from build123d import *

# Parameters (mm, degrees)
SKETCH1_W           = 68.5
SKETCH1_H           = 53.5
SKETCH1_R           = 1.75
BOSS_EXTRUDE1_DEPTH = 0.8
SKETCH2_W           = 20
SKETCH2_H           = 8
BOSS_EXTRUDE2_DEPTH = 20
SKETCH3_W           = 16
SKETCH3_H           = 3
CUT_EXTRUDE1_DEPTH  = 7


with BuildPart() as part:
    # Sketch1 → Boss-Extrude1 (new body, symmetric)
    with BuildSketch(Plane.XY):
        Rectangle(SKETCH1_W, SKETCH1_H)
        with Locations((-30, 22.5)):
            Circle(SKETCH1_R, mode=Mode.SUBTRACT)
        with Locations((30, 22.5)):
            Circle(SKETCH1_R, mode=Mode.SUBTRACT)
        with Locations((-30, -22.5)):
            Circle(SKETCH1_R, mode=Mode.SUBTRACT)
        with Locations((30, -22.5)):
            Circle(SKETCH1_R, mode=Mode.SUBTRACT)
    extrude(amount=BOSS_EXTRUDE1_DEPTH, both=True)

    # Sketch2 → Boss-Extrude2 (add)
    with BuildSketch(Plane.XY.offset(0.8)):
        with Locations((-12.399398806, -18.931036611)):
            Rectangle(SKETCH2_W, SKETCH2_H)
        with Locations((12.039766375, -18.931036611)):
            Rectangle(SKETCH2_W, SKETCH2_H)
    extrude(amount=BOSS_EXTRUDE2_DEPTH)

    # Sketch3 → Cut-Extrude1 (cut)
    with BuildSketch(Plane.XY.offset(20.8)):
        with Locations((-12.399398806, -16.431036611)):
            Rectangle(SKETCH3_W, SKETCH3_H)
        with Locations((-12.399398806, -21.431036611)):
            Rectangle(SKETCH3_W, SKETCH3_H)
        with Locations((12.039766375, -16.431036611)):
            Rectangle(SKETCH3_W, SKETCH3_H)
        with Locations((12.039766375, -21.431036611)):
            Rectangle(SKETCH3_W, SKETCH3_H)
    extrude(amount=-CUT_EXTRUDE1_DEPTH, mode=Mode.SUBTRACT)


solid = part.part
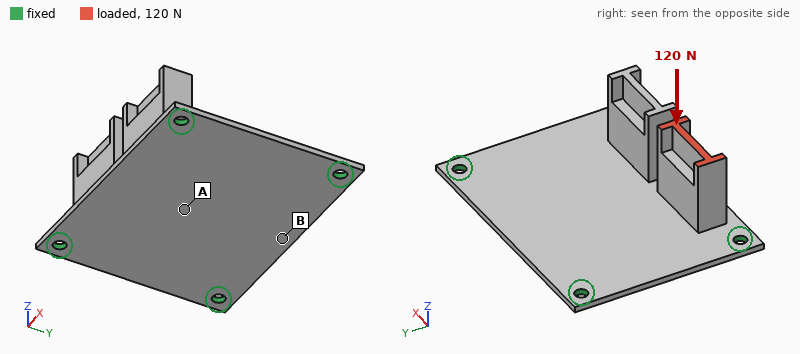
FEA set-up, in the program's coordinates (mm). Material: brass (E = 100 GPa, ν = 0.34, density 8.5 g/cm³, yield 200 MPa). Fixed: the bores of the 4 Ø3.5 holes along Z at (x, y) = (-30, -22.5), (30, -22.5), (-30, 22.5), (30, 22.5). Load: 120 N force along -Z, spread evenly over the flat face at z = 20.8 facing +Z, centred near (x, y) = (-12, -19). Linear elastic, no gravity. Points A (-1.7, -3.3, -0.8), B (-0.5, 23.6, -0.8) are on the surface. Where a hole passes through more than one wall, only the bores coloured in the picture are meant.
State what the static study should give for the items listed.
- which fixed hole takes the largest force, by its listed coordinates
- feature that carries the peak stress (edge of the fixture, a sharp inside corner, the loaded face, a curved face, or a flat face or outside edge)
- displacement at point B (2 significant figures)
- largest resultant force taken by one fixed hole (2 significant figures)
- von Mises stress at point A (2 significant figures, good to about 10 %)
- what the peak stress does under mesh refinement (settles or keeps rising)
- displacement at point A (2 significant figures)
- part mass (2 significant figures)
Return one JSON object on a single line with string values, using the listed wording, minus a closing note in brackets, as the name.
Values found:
{"which fixed hole takes the largest force, by its listed coordinates": "(-30, -22.5)", "feature that carries the peak stress": "edge of the fixture", "displacement at point B": "12 µm", "largest resultant force taken by one fixed hole": "90 N", "von Mises stress at point A": "17 MPa", "what the peak stress does under mesh refinement": "keeps rising", "displacement at point A": "45 µm", "part mass": "92 g"}
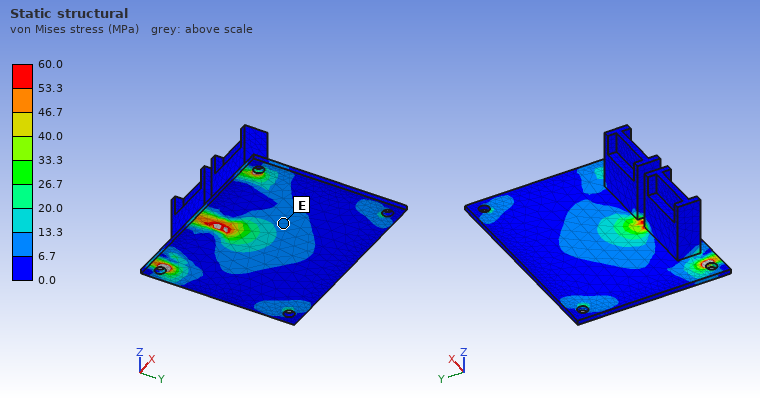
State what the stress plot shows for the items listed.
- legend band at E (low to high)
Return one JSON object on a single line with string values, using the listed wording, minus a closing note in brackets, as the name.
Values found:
{"legend band at E": "6.7 to 13.3 MPa"}
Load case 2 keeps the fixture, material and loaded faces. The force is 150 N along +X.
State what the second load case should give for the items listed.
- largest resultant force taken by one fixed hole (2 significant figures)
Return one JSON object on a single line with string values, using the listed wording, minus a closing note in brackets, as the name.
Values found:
{"largest resultant force taken by one fixed hole": "88 N"}
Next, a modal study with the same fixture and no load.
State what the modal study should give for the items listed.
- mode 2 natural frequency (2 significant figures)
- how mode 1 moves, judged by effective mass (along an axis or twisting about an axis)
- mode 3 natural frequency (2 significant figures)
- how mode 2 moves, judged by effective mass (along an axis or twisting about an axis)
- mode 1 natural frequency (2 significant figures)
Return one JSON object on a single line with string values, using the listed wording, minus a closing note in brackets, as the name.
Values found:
{"mode 2 natural frequency": "1300 Hz", "how mode 1 moves, judged by effective mass": "along Z", "mode 3 natural frequency": "2000 Hz", "how mode 2 moves, judged by effective mass": "along Y", "mode 1 natural frequency": "930 Hz"}
